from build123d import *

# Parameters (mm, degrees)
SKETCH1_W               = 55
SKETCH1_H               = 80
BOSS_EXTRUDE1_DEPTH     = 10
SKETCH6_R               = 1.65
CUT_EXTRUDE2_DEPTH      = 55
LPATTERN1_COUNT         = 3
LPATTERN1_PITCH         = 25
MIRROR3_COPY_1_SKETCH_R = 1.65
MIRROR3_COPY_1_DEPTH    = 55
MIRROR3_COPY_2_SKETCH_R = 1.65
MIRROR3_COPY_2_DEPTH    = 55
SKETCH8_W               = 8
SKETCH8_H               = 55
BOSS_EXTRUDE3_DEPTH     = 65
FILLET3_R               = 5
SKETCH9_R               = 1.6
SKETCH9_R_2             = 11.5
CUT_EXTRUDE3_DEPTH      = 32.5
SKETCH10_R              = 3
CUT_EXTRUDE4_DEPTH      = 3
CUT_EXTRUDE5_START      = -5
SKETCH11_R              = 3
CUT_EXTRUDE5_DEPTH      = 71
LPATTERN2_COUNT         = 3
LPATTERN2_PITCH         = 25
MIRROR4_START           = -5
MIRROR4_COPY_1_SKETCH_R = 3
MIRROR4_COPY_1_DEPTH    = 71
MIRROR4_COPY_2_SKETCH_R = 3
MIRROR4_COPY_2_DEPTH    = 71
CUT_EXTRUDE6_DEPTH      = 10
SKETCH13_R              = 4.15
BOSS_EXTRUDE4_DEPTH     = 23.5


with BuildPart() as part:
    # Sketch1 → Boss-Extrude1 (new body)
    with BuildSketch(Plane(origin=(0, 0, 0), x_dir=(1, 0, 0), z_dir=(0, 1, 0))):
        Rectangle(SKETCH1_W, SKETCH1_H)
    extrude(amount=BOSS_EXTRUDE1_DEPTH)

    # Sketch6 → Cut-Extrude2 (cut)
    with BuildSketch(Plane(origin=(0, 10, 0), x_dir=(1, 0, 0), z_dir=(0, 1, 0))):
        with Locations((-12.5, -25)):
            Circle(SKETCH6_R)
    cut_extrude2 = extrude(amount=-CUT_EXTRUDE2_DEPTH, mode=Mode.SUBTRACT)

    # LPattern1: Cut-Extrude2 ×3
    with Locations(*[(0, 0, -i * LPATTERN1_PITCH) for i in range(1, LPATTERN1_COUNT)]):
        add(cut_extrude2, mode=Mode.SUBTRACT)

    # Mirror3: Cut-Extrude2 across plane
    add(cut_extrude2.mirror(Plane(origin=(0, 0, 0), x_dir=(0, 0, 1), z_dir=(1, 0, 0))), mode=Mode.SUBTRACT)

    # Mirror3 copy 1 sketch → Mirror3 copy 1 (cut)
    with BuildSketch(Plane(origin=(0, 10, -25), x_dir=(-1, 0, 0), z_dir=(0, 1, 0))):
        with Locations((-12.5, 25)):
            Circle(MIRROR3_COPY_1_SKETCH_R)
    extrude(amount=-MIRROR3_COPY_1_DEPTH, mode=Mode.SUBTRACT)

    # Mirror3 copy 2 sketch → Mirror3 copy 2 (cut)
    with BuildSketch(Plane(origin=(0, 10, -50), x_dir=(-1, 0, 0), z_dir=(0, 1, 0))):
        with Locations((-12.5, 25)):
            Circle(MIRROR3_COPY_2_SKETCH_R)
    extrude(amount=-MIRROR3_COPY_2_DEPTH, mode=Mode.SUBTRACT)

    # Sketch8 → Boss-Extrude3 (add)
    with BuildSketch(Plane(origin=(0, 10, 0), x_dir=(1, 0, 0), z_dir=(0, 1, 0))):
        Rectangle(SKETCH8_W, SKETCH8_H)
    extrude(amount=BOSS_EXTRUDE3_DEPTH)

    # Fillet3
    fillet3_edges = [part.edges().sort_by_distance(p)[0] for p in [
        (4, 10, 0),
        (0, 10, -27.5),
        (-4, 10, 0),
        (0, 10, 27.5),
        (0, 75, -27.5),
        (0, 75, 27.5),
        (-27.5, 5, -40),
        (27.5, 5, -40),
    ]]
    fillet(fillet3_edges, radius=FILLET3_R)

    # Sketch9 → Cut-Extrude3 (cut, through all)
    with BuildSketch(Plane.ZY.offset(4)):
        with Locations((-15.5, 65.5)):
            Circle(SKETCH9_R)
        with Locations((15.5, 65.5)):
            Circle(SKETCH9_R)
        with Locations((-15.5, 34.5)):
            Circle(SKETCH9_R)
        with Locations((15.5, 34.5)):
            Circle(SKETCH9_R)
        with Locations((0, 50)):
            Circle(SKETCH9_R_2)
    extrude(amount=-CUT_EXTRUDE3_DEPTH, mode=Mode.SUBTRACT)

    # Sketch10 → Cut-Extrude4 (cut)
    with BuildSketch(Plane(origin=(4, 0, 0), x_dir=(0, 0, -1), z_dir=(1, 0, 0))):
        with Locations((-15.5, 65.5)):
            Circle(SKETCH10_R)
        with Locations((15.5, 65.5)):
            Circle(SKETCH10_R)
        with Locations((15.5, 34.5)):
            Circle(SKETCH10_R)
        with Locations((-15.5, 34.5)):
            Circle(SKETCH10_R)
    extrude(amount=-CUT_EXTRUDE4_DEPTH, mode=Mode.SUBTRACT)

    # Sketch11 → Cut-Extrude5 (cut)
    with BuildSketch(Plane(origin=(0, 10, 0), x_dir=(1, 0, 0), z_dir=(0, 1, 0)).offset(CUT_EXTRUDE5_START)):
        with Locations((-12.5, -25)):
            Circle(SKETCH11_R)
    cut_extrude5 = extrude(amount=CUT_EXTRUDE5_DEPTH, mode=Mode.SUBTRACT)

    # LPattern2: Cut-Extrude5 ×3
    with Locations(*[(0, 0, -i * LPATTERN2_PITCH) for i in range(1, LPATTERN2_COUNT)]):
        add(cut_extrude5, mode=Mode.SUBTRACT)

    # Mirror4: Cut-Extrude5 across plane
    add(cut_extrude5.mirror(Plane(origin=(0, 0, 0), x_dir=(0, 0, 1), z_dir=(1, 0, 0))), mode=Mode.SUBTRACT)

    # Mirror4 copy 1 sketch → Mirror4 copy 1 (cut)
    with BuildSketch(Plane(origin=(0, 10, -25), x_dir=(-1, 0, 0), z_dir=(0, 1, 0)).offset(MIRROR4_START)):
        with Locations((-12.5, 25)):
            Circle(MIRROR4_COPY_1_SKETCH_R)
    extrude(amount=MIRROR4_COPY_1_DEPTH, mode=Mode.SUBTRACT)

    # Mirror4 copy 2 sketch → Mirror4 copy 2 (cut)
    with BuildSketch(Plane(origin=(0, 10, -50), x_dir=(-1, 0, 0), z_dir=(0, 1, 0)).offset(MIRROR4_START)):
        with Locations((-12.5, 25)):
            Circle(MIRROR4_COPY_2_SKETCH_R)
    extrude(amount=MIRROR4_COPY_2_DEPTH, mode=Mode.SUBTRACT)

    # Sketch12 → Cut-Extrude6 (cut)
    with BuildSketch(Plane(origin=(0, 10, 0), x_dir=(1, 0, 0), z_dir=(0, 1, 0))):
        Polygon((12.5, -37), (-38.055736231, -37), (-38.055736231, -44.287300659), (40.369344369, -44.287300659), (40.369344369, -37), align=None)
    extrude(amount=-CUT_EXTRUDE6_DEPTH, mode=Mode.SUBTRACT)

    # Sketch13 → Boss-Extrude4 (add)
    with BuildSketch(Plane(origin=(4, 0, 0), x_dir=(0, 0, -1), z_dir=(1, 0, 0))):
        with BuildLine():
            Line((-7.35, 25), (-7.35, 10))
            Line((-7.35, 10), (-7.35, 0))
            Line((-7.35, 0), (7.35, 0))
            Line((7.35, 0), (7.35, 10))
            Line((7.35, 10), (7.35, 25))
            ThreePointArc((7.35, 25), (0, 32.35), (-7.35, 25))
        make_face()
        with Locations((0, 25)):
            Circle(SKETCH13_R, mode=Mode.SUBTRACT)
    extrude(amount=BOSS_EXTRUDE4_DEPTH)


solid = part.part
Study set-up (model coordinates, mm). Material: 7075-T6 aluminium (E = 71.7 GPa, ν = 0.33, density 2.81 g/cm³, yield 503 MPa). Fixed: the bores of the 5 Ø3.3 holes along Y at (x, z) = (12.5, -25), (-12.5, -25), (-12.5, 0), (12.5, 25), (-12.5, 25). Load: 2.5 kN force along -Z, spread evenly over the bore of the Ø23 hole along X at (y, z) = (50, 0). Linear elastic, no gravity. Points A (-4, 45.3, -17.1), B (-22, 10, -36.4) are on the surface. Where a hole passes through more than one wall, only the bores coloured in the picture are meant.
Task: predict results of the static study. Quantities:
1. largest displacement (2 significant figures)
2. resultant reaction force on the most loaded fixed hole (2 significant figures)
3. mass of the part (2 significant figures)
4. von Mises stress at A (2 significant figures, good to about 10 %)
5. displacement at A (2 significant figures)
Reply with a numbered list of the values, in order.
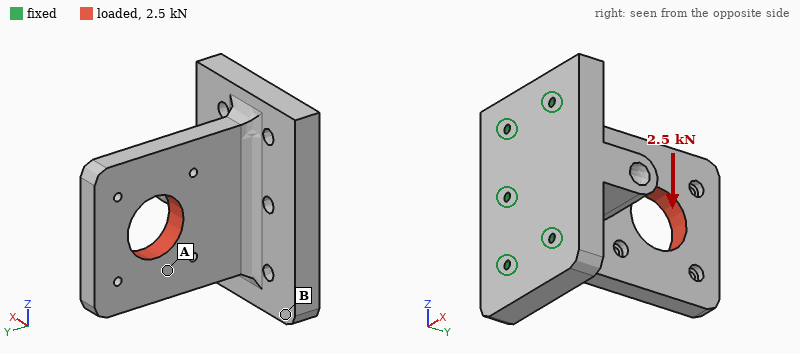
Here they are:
1. 46 µm
2. 1.4 kN
3. 200 g
4. 15 MPa
5. 24 µm
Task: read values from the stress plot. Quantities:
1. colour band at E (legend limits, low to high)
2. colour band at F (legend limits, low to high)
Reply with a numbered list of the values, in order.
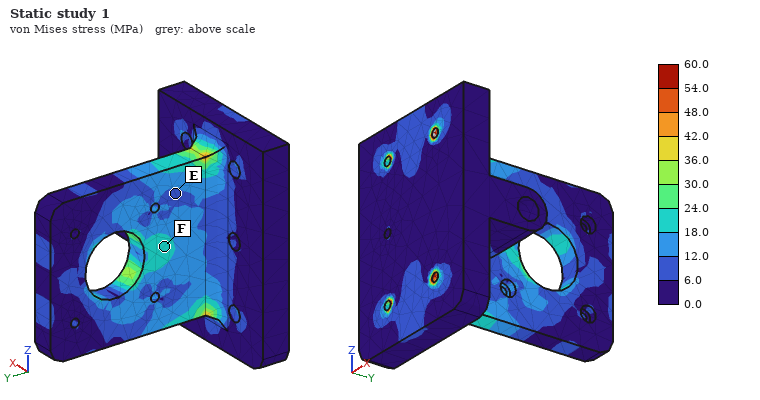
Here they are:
1. 6.0 to 12.0 MPa
2. 18.0 to 24.0 MPa
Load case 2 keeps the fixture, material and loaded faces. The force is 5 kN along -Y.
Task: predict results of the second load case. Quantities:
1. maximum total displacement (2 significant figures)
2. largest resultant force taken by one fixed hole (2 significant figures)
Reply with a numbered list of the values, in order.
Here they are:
1. 19 µm
2. 1.3 kN
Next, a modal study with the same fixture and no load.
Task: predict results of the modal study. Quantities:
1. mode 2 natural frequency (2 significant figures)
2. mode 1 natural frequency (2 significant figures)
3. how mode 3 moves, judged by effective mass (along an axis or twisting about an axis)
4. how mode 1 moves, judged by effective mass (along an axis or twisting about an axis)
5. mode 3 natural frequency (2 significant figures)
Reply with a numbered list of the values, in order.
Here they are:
1. 3900 Hz
2. 1900 Hz
3. along Z
4. along X
5. 5900 Hz
